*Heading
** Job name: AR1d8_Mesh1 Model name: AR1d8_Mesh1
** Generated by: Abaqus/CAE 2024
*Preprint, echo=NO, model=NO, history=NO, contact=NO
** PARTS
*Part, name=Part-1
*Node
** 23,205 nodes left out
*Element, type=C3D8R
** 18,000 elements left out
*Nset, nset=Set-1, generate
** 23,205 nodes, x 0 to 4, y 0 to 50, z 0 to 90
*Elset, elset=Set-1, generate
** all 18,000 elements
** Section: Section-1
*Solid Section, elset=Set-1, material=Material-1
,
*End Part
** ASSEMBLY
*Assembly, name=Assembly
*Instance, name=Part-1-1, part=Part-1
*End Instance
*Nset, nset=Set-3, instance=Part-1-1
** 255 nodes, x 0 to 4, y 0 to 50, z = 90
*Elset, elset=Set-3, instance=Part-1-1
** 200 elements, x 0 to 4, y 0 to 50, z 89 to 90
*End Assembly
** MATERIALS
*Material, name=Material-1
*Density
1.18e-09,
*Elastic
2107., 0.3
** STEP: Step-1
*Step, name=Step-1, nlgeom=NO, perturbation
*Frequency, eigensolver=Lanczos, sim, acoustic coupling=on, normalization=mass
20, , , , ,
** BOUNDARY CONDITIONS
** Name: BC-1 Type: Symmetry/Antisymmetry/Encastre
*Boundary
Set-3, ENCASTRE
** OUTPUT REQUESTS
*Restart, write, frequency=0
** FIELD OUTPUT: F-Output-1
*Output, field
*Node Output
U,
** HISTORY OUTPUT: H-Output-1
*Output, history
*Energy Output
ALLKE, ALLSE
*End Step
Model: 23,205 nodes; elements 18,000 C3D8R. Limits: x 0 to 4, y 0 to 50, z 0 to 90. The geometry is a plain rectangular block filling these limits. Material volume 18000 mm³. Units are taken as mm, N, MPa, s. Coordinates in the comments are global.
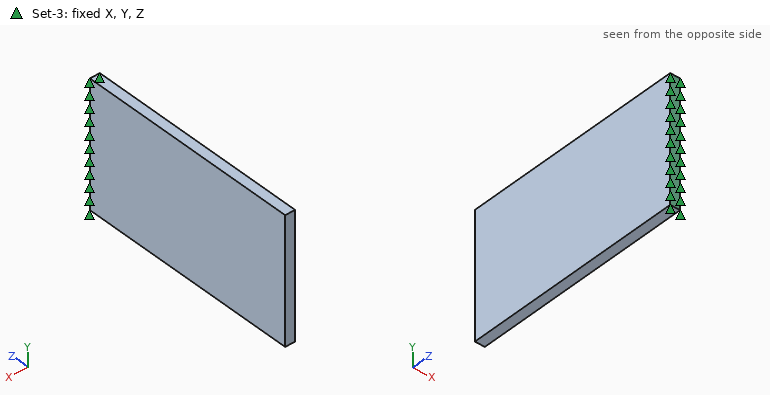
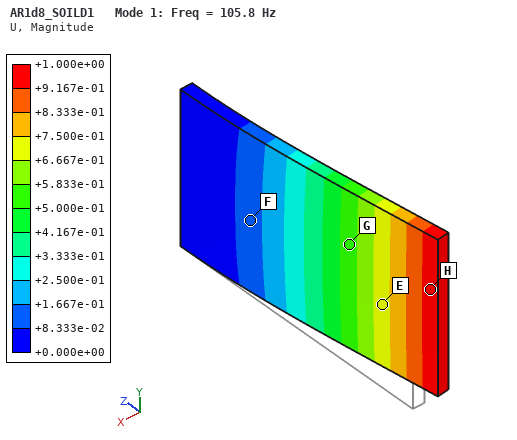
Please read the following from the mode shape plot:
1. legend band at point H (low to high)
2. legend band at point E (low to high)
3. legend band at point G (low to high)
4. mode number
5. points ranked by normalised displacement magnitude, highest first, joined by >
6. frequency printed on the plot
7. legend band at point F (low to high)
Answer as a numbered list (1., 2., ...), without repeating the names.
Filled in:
1. +9.167e-01 to +1.000e+00
2. +6.667e-01 to +7.500e-01
3. +5.000e-01 to +5.833e-01
4. 1
5. H > E > G > F
6. 105.8 Hz
7. +8.333e-02 to +1.667e-01
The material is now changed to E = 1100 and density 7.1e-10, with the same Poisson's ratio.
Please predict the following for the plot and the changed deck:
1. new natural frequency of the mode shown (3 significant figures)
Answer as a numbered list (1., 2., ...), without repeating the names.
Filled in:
1. 98.6 Hz
